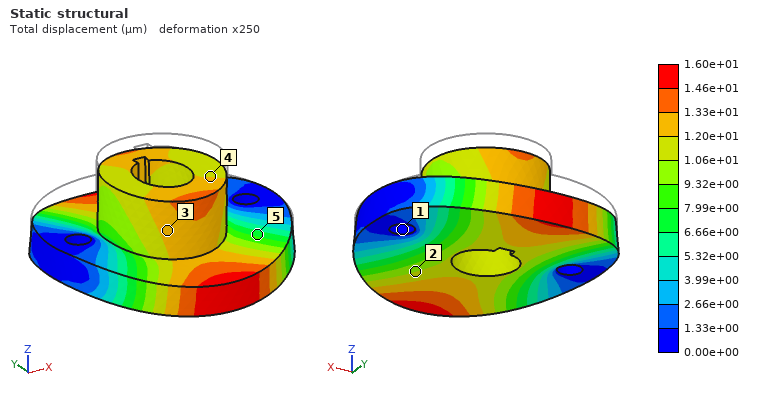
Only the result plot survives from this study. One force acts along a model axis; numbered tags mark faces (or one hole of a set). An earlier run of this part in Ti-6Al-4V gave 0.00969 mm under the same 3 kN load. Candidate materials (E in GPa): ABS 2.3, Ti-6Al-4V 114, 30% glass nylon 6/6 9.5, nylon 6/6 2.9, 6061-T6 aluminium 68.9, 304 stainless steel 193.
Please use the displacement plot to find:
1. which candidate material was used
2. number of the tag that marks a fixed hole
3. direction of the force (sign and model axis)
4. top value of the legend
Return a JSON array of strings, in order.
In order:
["6061-T6 aluminium", "1", "-Z", "1.60e+01 µm"]
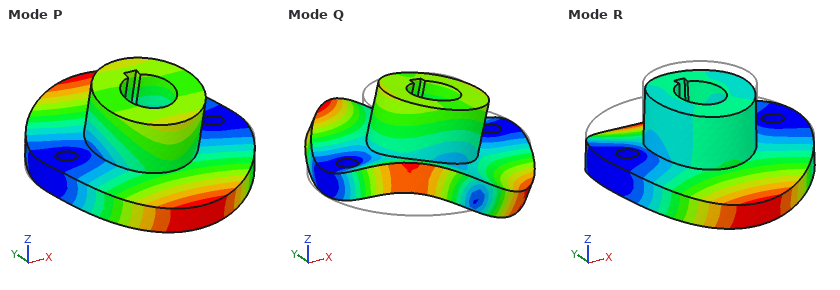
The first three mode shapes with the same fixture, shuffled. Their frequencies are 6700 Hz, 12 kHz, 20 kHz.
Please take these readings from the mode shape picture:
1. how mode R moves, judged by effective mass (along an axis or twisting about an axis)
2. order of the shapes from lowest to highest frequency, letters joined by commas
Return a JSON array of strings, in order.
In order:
["along Z", "P, R, Q"]
